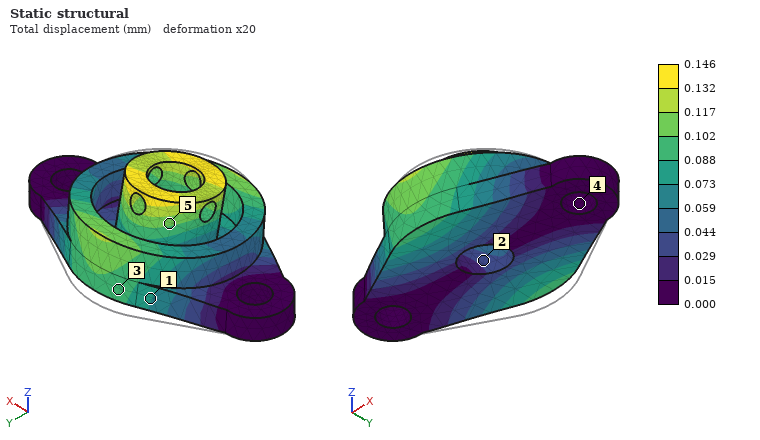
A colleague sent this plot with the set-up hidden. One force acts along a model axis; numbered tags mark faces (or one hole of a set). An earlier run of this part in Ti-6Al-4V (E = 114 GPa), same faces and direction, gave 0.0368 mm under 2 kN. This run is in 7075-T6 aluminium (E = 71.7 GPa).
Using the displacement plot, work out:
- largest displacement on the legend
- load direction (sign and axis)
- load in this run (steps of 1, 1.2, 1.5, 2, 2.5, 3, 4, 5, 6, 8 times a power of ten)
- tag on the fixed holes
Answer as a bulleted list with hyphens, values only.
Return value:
- 0.146 mm
- -Y
- 5 kN
- 4
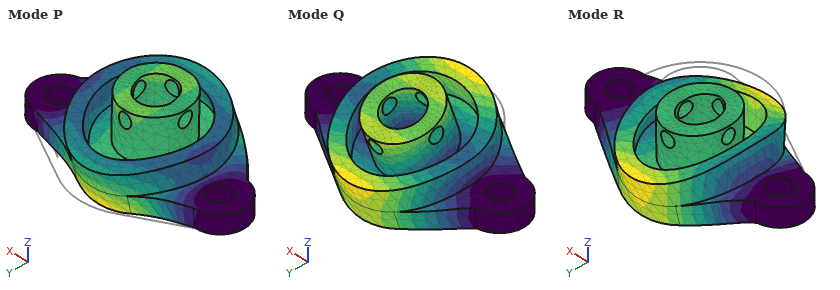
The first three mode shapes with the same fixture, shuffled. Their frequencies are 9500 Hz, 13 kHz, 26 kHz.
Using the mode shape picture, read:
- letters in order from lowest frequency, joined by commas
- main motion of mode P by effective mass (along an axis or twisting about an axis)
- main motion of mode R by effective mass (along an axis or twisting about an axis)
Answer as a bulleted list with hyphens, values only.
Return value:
- Q, R, P
- along Y
- along Z
